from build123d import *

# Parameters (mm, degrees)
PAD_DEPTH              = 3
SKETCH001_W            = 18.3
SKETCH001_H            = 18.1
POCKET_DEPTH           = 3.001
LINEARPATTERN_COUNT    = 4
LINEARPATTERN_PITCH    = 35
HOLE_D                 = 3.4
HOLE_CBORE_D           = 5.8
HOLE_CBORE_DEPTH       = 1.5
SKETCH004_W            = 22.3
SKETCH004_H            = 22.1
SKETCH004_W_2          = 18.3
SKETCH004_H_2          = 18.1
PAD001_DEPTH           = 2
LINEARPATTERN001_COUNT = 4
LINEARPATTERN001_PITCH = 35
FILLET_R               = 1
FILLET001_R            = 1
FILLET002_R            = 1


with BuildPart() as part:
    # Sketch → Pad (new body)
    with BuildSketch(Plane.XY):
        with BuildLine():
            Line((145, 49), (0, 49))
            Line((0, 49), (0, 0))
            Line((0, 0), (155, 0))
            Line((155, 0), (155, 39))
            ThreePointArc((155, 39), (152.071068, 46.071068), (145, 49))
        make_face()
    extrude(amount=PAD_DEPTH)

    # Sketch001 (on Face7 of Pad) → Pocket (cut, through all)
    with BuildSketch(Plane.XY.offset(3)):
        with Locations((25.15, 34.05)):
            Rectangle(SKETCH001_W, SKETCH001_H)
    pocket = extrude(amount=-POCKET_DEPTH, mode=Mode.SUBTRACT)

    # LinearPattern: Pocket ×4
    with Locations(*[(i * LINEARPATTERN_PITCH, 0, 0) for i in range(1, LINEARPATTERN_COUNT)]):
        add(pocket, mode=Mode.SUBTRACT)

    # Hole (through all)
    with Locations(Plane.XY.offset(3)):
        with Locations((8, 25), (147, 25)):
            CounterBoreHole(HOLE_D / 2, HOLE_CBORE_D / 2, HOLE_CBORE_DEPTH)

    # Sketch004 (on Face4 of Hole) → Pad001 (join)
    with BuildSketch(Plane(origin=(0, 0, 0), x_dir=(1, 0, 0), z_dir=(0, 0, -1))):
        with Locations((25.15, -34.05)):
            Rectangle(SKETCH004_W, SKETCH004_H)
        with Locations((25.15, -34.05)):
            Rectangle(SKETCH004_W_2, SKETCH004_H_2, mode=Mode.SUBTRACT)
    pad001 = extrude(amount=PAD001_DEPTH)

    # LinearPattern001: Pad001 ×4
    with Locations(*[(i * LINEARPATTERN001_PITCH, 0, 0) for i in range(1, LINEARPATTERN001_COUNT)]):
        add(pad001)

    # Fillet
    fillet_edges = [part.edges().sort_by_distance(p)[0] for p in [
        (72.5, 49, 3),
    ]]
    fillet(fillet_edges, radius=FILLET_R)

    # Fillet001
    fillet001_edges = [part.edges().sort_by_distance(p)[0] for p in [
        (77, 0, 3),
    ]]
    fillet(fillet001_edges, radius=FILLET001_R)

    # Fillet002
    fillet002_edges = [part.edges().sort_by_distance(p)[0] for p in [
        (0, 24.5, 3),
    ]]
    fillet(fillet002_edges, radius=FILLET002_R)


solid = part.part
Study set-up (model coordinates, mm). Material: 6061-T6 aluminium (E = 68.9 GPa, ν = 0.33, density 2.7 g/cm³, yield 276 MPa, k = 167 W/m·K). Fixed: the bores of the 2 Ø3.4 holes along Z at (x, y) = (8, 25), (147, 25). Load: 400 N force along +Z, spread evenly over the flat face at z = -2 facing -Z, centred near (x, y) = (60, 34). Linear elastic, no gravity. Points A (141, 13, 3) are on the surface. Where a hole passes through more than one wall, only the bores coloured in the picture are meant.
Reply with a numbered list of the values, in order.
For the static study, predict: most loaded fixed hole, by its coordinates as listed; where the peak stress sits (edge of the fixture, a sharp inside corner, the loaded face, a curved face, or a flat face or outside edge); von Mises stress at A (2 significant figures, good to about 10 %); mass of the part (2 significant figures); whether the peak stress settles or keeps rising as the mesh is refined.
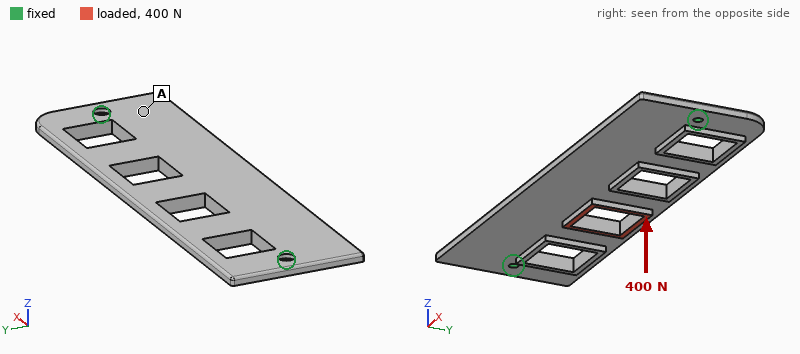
1. (8, 25)
2. edge of the fixture
3. 44 MPa
4. 54 g
5. keeps rising
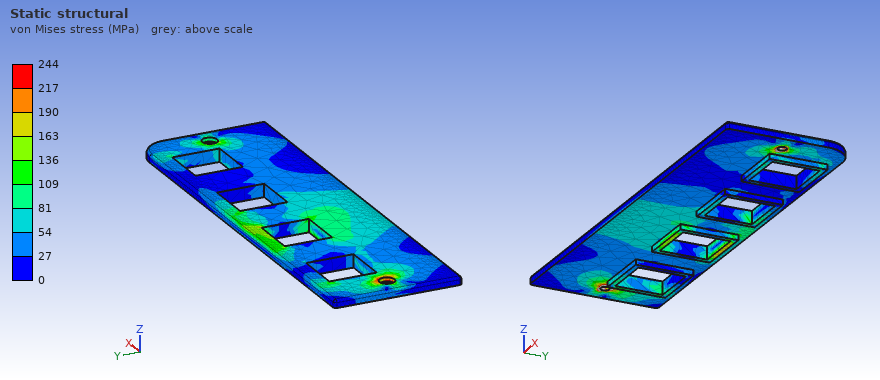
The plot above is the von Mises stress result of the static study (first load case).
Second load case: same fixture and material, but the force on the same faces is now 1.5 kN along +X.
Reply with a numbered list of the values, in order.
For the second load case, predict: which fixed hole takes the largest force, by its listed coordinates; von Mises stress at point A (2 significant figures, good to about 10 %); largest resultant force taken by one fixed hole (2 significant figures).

1. (8, 25)
2. 14 MPa
3. 930 N
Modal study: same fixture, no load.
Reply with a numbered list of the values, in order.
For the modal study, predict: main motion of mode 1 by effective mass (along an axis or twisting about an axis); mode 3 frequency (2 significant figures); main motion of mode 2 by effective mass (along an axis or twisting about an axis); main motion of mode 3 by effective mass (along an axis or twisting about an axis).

1. along Z
2. 1700 Hz
3. twisting about X
4. twisting about Y
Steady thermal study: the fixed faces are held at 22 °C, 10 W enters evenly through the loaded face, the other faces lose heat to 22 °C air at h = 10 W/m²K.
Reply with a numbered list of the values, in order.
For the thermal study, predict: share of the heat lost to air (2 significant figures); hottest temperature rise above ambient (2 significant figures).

1. 16 %
2. 23 K
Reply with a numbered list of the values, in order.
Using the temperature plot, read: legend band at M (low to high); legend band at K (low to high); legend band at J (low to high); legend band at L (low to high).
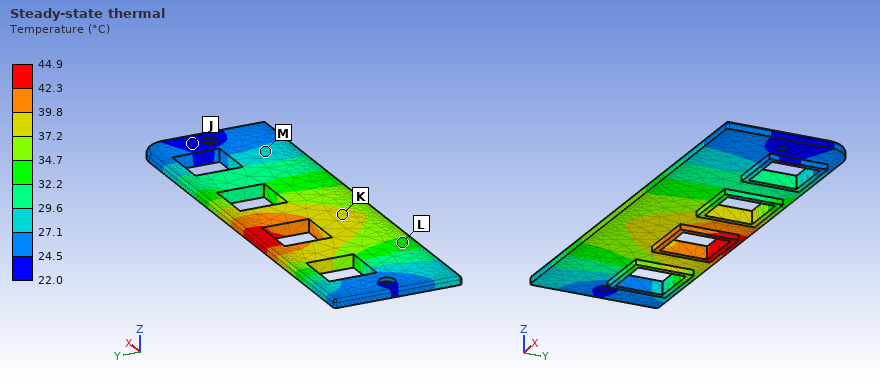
1. 27.1 to 29.6 °C
2. 37.2 to 39.8 °C
3. 22.0 to 24.5 °C
4. 32.2 to 34.7 °C
